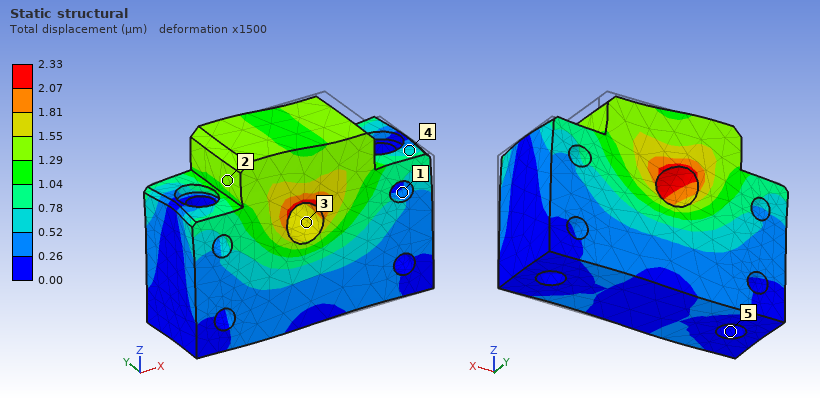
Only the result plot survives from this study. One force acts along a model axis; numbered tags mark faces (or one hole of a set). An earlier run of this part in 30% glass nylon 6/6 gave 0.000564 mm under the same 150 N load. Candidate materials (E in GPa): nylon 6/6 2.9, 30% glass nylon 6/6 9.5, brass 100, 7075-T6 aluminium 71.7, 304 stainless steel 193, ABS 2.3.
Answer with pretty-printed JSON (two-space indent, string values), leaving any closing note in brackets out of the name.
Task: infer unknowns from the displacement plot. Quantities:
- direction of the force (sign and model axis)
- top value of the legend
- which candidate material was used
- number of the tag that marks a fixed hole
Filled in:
{
  "direction of the force": "-X",
  "top value of the legend": "2.33 µm",
  "which candidate material was used": "ABS",
  "number of the tag that marks a fixed hole": "5"
}
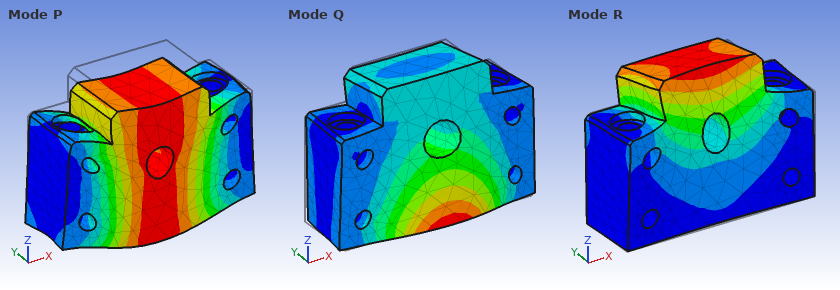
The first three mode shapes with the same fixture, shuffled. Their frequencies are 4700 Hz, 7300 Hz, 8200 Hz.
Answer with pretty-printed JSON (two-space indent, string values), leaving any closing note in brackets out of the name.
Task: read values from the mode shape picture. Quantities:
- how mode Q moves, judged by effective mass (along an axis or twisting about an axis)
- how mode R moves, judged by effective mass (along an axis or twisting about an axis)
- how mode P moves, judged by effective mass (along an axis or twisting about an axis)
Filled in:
{
  "how mode Q moves, judged by effective mass": "along Y",
  "how mode R moves, judged by effective mass": "along Y",
  "how mode P moves, judged by effective mass": "along Z"
}
